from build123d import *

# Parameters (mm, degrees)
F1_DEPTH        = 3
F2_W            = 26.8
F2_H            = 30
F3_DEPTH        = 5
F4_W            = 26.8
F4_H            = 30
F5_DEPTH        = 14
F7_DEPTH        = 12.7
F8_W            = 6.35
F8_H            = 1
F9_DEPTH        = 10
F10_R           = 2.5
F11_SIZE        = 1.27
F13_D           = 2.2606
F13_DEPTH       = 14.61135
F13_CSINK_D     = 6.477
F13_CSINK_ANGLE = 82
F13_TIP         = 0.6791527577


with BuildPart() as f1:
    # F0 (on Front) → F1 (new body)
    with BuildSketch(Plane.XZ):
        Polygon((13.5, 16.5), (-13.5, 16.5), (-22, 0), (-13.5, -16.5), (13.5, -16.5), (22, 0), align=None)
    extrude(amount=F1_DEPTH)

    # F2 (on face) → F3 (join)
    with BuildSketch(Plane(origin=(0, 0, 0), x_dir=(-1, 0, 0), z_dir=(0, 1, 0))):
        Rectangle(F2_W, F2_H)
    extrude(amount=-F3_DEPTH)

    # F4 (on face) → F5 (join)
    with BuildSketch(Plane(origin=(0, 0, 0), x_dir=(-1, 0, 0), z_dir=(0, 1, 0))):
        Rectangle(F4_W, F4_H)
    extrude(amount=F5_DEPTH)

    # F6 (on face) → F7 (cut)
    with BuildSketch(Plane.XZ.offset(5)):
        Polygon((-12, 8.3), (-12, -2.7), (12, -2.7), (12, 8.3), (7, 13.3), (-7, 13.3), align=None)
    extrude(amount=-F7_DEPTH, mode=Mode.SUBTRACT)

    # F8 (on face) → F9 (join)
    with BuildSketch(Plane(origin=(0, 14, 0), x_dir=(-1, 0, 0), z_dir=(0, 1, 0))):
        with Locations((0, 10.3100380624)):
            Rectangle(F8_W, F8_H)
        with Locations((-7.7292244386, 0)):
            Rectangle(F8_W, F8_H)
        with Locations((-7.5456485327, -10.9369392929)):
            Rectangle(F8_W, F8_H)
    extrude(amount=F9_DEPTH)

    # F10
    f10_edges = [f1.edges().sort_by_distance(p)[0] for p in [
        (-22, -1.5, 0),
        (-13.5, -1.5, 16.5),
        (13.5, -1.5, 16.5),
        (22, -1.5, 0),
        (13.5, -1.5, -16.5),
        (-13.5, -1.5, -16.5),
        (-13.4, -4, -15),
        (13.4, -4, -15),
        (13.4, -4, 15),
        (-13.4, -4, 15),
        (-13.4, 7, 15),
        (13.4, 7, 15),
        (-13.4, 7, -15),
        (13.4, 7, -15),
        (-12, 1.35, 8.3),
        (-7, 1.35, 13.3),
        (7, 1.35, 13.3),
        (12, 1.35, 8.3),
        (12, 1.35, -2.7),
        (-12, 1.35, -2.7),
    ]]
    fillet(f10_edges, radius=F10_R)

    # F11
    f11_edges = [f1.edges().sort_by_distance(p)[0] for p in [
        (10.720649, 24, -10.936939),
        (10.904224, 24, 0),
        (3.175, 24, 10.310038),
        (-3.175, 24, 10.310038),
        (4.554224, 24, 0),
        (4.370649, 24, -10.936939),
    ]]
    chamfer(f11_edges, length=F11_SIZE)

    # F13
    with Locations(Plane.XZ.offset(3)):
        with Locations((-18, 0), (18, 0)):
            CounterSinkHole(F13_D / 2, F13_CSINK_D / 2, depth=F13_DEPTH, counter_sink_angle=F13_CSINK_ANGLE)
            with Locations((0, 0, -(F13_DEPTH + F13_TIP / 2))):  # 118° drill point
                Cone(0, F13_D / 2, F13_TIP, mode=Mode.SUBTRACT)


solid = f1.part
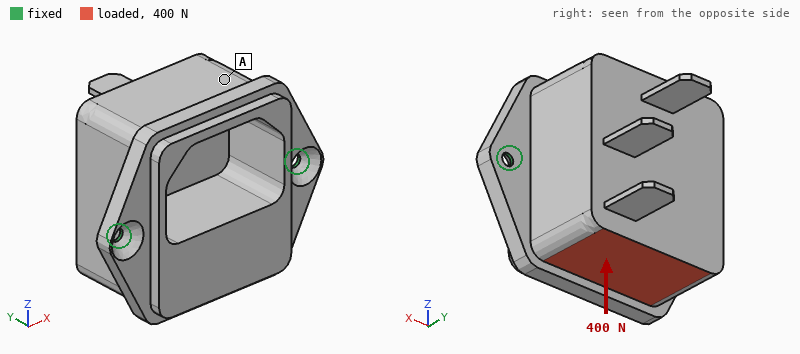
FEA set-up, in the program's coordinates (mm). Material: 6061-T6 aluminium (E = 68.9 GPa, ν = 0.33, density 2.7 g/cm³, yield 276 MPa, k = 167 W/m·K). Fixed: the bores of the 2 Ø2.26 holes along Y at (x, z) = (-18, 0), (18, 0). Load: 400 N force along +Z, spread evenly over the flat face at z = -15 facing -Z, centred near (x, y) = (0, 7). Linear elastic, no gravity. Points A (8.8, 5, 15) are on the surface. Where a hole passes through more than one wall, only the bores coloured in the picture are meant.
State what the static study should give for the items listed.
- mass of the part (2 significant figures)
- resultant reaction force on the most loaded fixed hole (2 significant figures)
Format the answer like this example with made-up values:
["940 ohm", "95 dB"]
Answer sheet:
["32 g", "200 N"]
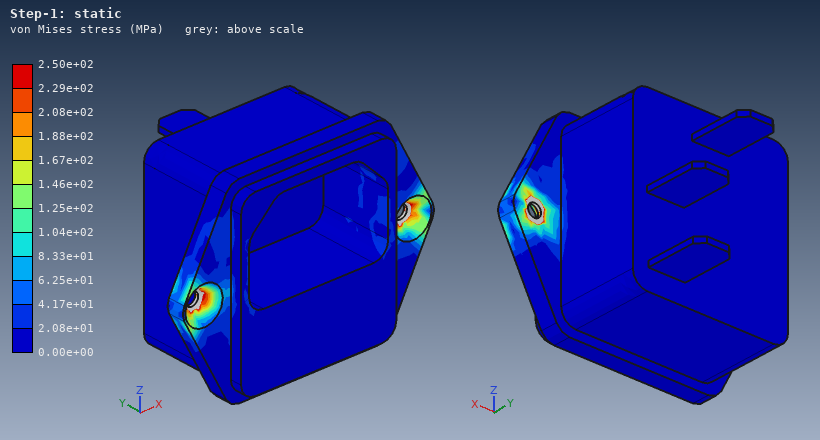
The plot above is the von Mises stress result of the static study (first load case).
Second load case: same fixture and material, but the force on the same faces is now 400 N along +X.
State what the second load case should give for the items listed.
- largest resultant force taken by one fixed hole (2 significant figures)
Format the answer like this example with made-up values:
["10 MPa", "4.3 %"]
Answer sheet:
["270 N"]
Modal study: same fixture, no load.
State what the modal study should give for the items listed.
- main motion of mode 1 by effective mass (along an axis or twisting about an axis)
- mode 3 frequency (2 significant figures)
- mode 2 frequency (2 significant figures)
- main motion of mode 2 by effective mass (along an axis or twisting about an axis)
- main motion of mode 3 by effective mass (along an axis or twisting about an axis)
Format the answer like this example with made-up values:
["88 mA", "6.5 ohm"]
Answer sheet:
["along Z", "6600 Hz", "5800 Hz", "along Y", "along X"]
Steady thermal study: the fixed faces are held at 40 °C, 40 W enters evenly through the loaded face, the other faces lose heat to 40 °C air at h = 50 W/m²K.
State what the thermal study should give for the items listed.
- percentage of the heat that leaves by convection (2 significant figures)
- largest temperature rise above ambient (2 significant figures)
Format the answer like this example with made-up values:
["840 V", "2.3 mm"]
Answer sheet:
["21 %", "42 K"]
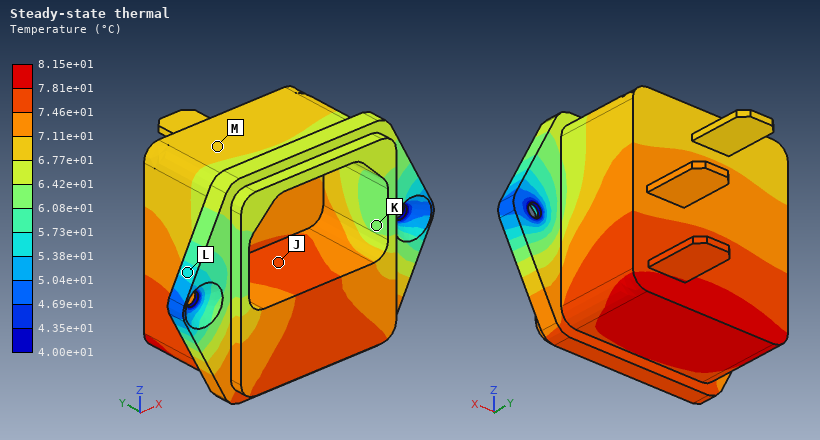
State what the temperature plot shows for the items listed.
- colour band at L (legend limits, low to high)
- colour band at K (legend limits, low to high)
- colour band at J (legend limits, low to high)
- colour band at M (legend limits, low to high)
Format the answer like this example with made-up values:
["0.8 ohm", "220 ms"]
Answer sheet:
["5.38e+01 to 5.73e+01 °C", "6.08e+01 to 6.42e+01 °C", "7.46e+01 to 7.81e+01 °C", "6.77e+01 to 7.11e+01 °C"]
